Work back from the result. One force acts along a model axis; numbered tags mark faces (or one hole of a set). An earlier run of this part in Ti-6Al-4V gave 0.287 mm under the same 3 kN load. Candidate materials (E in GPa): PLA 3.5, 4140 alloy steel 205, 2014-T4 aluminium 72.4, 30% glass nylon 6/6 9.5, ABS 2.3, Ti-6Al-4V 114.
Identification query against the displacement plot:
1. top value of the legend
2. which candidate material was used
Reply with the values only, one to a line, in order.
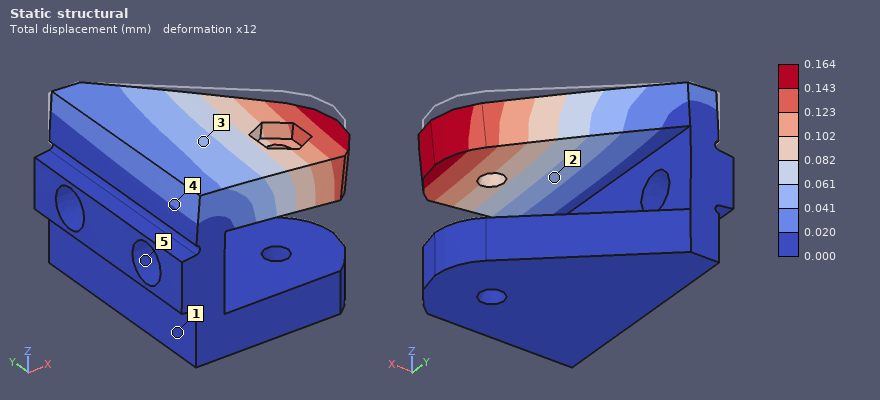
0.164 mm
4140 alloy steel
